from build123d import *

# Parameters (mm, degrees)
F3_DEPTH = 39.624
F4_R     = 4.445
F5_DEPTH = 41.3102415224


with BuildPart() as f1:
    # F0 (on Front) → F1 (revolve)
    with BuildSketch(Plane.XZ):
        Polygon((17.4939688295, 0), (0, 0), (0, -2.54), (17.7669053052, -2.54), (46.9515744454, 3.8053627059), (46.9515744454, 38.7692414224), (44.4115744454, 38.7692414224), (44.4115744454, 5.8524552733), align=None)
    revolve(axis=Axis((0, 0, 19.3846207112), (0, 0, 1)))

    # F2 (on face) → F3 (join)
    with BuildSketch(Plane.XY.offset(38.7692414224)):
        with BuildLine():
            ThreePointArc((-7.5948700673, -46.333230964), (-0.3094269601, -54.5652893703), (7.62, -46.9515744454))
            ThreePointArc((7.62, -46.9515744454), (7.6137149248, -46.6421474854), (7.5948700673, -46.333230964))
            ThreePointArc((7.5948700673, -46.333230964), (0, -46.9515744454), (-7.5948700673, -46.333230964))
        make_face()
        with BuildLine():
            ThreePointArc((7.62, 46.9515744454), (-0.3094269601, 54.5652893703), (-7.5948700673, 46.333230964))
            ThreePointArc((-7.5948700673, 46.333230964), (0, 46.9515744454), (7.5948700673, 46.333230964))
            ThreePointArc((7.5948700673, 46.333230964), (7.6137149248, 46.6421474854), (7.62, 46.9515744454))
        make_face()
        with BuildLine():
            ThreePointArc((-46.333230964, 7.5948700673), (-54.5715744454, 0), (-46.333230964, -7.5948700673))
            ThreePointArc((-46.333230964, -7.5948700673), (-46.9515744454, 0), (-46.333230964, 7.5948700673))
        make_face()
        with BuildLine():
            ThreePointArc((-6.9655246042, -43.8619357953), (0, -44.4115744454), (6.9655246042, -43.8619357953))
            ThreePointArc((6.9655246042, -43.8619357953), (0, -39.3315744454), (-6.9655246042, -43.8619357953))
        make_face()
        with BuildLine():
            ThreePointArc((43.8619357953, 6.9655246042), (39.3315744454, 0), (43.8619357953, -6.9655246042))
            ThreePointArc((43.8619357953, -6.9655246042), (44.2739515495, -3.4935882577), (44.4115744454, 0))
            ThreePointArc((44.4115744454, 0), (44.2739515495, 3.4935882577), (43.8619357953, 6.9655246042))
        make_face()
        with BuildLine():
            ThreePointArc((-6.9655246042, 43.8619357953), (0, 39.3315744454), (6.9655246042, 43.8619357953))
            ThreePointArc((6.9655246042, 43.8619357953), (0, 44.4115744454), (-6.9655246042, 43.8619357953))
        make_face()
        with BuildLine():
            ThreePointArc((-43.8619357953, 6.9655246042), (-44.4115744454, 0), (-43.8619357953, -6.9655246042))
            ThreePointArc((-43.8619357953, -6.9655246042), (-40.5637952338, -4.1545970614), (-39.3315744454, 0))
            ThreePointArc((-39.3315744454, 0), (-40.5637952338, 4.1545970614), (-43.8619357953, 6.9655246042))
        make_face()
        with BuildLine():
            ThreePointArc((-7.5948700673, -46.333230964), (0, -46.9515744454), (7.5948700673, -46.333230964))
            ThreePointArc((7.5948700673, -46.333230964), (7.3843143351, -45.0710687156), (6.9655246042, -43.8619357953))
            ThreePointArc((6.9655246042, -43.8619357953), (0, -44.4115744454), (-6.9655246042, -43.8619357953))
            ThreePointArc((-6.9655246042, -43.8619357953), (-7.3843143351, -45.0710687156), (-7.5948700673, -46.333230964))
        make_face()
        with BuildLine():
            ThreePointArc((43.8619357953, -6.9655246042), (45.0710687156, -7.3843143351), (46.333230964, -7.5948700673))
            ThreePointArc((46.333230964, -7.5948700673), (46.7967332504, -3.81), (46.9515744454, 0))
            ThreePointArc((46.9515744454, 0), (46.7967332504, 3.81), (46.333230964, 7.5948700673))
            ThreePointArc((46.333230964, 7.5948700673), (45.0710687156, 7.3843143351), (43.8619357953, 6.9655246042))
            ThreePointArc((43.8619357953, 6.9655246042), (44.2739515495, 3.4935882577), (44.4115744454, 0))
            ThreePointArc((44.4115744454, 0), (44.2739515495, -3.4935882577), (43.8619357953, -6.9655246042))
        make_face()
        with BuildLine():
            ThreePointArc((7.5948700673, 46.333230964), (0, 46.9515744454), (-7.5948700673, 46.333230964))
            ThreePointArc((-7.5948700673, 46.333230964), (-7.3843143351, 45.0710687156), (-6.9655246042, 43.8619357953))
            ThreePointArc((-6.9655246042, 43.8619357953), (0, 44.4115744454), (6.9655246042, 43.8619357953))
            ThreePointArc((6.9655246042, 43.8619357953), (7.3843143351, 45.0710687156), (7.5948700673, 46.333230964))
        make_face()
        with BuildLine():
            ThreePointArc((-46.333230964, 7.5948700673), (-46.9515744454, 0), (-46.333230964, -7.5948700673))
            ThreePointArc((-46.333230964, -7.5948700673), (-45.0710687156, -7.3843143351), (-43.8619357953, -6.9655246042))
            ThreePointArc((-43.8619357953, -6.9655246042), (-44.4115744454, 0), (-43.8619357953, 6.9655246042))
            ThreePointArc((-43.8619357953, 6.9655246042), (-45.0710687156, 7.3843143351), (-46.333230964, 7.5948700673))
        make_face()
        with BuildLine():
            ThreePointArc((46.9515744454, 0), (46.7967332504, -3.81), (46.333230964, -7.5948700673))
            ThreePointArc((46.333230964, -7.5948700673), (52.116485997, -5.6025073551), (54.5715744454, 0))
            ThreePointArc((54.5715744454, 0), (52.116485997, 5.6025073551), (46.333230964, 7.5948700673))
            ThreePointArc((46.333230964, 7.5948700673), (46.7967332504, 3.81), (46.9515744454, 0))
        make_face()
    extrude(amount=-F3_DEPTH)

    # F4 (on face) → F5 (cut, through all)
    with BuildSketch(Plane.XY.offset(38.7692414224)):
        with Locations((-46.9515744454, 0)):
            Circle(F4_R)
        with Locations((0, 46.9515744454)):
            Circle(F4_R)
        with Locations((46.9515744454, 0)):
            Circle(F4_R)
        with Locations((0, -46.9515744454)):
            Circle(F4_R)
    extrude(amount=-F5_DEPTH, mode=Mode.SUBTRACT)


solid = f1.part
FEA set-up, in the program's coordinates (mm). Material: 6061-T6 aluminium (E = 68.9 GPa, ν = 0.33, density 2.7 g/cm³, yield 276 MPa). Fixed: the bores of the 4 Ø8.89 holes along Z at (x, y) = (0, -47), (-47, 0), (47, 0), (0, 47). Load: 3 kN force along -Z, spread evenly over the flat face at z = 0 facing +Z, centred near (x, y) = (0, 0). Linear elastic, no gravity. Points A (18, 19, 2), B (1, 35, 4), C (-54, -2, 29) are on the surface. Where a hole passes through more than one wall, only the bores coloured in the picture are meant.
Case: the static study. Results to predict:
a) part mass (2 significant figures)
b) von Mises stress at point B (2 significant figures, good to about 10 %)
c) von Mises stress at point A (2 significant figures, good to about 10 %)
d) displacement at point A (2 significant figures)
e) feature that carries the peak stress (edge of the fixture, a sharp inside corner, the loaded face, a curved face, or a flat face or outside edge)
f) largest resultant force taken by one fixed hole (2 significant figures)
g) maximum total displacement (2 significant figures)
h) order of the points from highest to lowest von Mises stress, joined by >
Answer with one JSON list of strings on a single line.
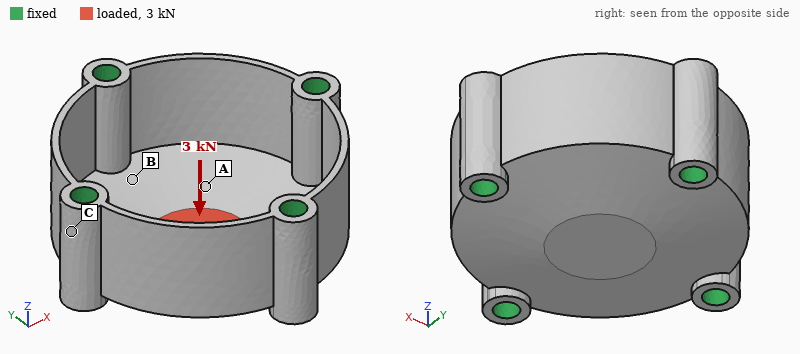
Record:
["150 g", "91 MPa", "56 MPa", "0.054 mm", "a flat face or outside edge", "2.5 kN", "0.25 mm", "B > A > C"]
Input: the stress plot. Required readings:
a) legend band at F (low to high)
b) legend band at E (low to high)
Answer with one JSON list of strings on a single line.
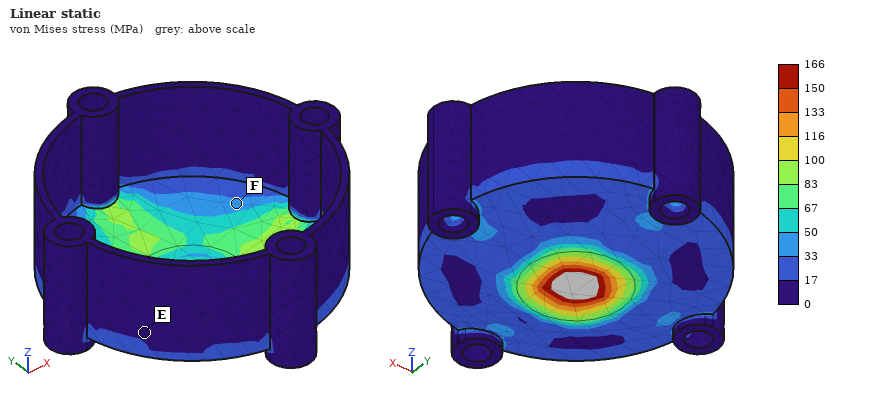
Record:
["33 to 50 MPa", "0 to 17 MPa"]
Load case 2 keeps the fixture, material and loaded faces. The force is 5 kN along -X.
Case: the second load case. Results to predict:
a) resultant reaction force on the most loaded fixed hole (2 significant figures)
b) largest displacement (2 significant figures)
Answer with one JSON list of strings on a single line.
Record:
["1.4 kN", "49 µm"]
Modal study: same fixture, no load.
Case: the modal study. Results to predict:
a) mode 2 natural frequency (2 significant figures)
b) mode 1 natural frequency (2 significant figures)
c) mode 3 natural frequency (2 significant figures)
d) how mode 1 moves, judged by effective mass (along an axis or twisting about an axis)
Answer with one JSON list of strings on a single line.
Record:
["8300 Hz", "6500 Hz", "8300 Hz", "along Z"]
